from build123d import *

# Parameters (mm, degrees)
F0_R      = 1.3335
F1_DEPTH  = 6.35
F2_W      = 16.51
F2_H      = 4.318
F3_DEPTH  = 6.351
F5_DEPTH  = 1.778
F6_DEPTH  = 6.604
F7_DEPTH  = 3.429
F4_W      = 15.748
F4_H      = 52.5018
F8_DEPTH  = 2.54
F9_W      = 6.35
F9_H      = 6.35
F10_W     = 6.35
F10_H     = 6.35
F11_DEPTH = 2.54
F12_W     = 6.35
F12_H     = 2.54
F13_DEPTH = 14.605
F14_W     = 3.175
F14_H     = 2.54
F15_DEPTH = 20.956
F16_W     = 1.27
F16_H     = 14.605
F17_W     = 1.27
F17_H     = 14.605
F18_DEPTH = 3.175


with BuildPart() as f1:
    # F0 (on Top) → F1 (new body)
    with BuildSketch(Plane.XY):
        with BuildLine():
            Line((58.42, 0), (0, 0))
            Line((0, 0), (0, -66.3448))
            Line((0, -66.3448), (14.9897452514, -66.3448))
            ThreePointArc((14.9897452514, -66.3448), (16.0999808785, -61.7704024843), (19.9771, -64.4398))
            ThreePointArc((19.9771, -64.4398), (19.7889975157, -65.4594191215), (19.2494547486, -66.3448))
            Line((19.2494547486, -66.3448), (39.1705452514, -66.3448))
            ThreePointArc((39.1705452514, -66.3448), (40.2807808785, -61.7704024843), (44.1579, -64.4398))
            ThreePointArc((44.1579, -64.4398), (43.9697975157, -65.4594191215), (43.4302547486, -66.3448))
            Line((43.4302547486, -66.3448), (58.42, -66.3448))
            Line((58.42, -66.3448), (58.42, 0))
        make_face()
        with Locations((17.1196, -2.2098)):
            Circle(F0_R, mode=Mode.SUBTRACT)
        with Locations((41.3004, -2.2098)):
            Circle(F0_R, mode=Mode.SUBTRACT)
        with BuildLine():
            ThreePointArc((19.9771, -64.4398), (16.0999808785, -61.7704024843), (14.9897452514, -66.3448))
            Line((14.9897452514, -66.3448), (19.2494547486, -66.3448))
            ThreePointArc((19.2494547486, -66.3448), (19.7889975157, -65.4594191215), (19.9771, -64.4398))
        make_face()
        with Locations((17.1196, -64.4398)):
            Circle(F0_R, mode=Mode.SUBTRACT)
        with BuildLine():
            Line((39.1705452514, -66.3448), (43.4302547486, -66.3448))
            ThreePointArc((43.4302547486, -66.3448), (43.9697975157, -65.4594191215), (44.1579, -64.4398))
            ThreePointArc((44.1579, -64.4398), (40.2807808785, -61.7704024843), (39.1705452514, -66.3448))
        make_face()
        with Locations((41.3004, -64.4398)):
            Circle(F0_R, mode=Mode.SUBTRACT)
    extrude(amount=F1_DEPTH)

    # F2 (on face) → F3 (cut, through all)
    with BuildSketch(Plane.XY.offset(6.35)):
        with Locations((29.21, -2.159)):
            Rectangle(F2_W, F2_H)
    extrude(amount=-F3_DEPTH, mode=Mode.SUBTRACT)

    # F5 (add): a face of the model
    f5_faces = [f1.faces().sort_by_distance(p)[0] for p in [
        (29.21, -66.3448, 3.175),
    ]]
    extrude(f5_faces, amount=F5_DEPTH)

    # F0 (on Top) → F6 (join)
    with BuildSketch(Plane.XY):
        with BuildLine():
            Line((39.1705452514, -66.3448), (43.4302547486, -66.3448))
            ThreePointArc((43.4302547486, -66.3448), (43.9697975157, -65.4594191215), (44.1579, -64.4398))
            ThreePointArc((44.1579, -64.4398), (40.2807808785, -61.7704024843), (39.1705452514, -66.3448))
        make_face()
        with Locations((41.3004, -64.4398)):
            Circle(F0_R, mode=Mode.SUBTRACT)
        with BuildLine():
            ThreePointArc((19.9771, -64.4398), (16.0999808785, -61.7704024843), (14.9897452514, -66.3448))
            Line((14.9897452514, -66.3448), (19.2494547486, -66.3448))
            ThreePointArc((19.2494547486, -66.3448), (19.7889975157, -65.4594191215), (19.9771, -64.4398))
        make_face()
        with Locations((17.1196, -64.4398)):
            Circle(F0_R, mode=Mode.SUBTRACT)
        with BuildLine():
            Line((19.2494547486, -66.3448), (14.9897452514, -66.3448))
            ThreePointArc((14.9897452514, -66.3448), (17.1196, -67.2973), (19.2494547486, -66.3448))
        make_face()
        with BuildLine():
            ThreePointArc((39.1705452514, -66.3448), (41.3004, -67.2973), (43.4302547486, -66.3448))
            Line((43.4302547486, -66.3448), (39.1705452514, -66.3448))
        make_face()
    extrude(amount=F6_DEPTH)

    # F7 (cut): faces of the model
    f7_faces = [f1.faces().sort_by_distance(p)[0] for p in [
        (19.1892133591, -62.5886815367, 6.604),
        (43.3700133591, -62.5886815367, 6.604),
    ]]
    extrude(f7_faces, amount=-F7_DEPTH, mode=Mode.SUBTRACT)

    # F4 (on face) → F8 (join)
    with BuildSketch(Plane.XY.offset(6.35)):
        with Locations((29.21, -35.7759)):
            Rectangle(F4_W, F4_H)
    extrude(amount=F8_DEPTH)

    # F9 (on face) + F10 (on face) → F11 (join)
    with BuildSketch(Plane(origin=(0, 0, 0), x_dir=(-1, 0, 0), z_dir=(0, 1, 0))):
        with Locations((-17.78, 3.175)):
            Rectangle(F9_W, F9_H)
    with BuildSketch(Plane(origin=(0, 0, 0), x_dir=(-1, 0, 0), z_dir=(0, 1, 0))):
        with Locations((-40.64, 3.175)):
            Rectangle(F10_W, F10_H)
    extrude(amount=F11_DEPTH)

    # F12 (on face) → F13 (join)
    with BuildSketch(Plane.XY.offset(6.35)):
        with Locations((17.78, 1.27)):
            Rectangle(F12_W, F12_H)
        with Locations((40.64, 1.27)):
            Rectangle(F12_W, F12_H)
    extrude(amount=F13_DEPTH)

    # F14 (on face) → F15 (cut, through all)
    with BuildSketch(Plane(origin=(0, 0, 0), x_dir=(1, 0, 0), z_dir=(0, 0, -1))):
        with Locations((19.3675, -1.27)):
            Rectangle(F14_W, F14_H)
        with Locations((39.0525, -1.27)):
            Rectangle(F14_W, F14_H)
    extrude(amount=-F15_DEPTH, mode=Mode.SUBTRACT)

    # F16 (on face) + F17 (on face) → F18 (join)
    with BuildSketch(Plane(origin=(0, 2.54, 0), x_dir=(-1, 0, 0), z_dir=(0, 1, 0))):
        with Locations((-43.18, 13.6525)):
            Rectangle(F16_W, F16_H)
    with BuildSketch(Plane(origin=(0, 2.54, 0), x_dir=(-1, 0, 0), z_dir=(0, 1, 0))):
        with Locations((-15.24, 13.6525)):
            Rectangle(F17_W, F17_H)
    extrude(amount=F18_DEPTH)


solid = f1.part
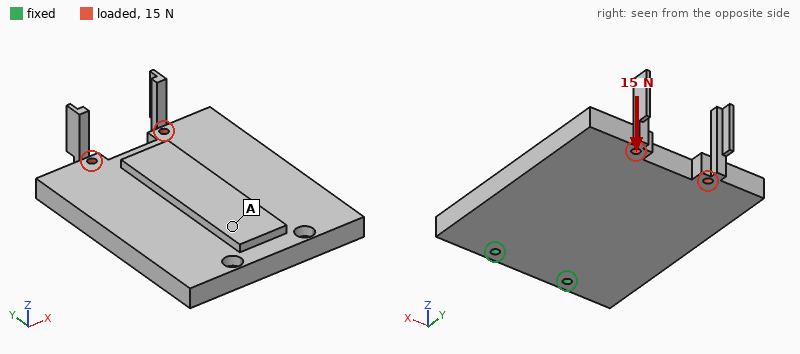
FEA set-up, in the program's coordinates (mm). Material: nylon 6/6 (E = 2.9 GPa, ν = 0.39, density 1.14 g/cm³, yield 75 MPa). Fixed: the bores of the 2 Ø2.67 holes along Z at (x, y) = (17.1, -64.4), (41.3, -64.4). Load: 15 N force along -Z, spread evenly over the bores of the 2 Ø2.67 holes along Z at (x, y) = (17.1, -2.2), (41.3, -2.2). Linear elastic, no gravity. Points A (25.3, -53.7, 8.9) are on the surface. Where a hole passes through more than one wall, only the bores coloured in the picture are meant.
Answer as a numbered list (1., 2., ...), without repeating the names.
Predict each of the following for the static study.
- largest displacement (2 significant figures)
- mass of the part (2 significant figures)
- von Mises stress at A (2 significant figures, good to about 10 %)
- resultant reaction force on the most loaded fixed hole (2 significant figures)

1. 0.88 mm
2. 31 g
3. 1.8 MPa
4. 7.6 N
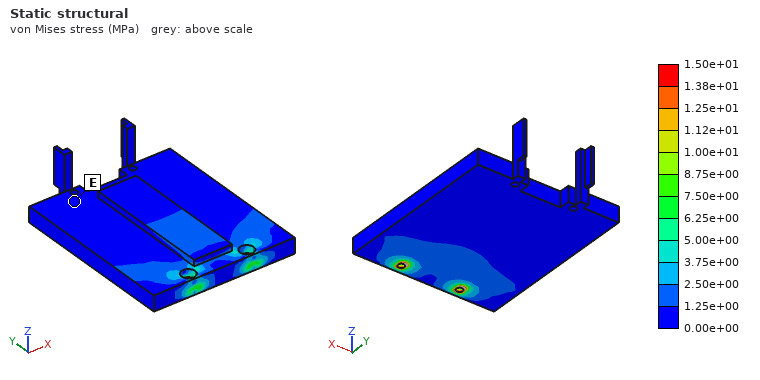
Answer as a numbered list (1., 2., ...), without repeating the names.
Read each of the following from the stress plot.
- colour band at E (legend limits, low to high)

1. 0.00e+00 to 1.25e+00 MPa
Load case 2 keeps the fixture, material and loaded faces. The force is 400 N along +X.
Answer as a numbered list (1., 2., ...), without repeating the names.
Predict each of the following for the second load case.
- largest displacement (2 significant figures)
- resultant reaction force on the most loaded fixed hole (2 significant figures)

1. 0.81 mm
2. 1000 N
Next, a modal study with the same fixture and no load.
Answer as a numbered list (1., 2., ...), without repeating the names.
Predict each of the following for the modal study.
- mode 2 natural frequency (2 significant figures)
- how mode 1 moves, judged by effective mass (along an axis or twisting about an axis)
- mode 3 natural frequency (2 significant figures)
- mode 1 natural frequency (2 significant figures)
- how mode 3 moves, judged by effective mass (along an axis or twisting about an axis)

1. 830 Hz
2. along Z
3. 1200 Hz
4. 230 Hz
5. along X
